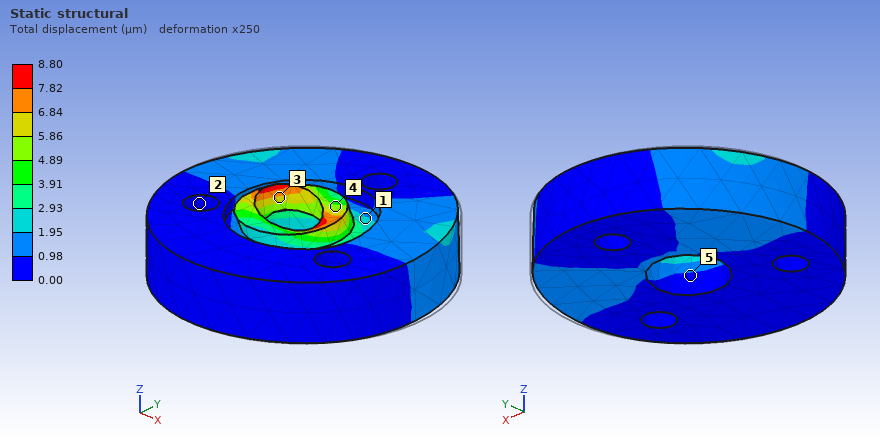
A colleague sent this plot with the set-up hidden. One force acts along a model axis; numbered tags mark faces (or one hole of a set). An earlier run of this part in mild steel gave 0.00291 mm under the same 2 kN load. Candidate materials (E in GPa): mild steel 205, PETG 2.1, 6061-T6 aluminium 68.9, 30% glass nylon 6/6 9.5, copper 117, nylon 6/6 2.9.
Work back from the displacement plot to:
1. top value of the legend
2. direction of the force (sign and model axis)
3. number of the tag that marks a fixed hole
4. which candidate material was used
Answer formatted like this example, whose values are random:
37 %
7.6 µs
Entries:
8.80 µm
-X
2
6061-T6 aluminium
